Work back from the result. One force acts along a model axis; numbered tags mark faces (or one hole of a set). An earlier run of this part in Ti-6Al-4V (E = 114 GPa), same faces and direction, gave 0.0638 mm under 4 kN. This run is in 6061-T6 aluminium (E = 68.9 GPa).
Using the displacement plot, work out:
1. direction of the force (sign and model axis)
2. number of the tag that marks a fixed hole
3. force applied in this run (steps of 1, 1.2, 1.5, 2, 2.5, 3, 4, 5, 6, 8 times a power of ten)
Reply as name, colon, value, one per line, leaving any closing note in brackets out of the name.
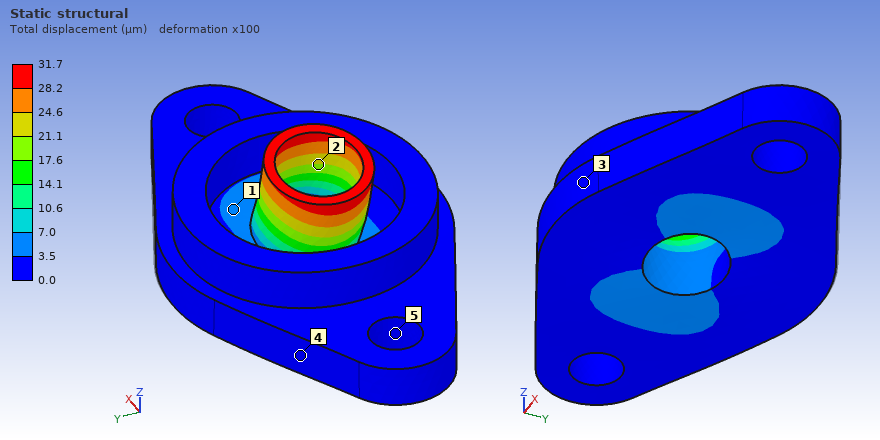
direction of the force: -X
number of the tag that marks a fixed hole: 5
force applied in this run: 1.2 kN
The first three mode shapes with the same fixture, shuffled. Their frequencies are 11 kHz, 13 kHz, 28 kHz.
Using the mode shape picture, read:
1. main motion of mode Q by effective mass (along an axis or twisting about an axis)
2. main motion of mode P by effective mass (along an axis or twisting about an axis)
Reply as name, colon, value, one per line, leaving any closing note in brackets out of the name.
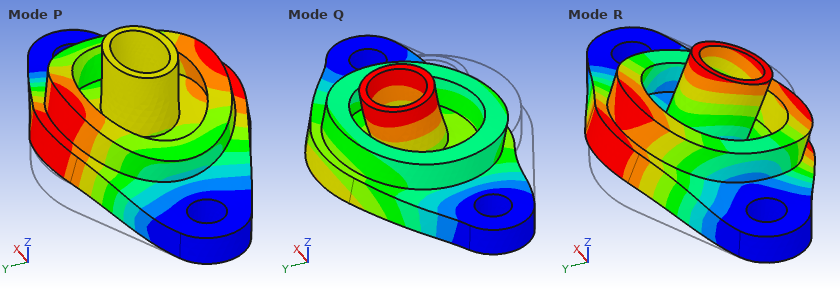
main motion of mode Q by effective mass: along Y
main motion of mode P by effective mass: along Z
